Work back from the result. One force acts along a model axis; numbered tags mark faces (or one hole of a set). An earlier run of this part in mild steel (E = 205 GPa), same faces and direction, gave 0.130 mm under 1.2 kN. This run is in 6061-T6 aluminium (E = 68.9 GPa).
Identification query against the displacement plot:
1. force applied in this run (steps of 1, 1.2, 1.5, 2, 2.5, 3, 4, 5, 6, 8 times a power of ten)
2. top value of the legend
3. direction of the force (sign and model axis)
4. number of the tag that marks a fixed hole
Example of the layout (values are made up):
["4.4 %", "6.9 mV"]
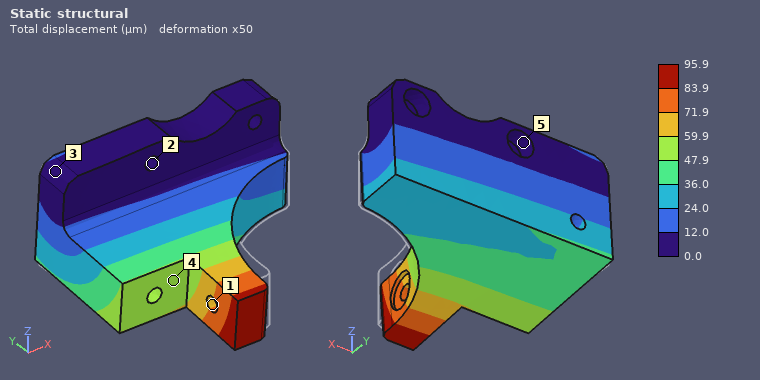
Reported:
["300 N", "95.9 µm", "-Z", "2"]
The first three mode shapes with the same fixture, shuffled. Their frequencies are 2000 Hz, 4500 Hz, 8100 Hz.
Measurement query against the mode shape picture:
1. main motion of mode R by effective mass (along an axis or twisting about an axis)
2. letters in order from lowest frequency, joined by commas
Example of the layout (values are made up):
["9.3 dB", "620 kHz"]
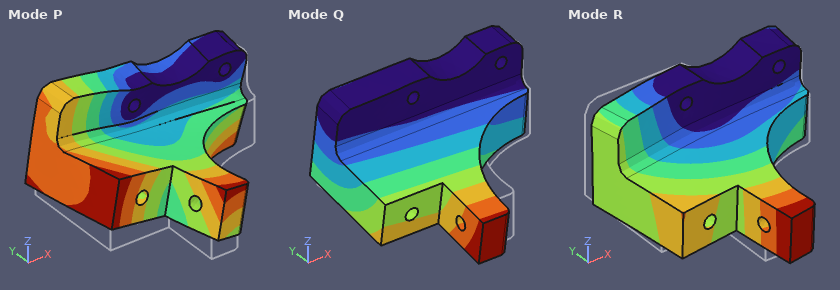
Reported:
["along X", "Q, R, P"]
